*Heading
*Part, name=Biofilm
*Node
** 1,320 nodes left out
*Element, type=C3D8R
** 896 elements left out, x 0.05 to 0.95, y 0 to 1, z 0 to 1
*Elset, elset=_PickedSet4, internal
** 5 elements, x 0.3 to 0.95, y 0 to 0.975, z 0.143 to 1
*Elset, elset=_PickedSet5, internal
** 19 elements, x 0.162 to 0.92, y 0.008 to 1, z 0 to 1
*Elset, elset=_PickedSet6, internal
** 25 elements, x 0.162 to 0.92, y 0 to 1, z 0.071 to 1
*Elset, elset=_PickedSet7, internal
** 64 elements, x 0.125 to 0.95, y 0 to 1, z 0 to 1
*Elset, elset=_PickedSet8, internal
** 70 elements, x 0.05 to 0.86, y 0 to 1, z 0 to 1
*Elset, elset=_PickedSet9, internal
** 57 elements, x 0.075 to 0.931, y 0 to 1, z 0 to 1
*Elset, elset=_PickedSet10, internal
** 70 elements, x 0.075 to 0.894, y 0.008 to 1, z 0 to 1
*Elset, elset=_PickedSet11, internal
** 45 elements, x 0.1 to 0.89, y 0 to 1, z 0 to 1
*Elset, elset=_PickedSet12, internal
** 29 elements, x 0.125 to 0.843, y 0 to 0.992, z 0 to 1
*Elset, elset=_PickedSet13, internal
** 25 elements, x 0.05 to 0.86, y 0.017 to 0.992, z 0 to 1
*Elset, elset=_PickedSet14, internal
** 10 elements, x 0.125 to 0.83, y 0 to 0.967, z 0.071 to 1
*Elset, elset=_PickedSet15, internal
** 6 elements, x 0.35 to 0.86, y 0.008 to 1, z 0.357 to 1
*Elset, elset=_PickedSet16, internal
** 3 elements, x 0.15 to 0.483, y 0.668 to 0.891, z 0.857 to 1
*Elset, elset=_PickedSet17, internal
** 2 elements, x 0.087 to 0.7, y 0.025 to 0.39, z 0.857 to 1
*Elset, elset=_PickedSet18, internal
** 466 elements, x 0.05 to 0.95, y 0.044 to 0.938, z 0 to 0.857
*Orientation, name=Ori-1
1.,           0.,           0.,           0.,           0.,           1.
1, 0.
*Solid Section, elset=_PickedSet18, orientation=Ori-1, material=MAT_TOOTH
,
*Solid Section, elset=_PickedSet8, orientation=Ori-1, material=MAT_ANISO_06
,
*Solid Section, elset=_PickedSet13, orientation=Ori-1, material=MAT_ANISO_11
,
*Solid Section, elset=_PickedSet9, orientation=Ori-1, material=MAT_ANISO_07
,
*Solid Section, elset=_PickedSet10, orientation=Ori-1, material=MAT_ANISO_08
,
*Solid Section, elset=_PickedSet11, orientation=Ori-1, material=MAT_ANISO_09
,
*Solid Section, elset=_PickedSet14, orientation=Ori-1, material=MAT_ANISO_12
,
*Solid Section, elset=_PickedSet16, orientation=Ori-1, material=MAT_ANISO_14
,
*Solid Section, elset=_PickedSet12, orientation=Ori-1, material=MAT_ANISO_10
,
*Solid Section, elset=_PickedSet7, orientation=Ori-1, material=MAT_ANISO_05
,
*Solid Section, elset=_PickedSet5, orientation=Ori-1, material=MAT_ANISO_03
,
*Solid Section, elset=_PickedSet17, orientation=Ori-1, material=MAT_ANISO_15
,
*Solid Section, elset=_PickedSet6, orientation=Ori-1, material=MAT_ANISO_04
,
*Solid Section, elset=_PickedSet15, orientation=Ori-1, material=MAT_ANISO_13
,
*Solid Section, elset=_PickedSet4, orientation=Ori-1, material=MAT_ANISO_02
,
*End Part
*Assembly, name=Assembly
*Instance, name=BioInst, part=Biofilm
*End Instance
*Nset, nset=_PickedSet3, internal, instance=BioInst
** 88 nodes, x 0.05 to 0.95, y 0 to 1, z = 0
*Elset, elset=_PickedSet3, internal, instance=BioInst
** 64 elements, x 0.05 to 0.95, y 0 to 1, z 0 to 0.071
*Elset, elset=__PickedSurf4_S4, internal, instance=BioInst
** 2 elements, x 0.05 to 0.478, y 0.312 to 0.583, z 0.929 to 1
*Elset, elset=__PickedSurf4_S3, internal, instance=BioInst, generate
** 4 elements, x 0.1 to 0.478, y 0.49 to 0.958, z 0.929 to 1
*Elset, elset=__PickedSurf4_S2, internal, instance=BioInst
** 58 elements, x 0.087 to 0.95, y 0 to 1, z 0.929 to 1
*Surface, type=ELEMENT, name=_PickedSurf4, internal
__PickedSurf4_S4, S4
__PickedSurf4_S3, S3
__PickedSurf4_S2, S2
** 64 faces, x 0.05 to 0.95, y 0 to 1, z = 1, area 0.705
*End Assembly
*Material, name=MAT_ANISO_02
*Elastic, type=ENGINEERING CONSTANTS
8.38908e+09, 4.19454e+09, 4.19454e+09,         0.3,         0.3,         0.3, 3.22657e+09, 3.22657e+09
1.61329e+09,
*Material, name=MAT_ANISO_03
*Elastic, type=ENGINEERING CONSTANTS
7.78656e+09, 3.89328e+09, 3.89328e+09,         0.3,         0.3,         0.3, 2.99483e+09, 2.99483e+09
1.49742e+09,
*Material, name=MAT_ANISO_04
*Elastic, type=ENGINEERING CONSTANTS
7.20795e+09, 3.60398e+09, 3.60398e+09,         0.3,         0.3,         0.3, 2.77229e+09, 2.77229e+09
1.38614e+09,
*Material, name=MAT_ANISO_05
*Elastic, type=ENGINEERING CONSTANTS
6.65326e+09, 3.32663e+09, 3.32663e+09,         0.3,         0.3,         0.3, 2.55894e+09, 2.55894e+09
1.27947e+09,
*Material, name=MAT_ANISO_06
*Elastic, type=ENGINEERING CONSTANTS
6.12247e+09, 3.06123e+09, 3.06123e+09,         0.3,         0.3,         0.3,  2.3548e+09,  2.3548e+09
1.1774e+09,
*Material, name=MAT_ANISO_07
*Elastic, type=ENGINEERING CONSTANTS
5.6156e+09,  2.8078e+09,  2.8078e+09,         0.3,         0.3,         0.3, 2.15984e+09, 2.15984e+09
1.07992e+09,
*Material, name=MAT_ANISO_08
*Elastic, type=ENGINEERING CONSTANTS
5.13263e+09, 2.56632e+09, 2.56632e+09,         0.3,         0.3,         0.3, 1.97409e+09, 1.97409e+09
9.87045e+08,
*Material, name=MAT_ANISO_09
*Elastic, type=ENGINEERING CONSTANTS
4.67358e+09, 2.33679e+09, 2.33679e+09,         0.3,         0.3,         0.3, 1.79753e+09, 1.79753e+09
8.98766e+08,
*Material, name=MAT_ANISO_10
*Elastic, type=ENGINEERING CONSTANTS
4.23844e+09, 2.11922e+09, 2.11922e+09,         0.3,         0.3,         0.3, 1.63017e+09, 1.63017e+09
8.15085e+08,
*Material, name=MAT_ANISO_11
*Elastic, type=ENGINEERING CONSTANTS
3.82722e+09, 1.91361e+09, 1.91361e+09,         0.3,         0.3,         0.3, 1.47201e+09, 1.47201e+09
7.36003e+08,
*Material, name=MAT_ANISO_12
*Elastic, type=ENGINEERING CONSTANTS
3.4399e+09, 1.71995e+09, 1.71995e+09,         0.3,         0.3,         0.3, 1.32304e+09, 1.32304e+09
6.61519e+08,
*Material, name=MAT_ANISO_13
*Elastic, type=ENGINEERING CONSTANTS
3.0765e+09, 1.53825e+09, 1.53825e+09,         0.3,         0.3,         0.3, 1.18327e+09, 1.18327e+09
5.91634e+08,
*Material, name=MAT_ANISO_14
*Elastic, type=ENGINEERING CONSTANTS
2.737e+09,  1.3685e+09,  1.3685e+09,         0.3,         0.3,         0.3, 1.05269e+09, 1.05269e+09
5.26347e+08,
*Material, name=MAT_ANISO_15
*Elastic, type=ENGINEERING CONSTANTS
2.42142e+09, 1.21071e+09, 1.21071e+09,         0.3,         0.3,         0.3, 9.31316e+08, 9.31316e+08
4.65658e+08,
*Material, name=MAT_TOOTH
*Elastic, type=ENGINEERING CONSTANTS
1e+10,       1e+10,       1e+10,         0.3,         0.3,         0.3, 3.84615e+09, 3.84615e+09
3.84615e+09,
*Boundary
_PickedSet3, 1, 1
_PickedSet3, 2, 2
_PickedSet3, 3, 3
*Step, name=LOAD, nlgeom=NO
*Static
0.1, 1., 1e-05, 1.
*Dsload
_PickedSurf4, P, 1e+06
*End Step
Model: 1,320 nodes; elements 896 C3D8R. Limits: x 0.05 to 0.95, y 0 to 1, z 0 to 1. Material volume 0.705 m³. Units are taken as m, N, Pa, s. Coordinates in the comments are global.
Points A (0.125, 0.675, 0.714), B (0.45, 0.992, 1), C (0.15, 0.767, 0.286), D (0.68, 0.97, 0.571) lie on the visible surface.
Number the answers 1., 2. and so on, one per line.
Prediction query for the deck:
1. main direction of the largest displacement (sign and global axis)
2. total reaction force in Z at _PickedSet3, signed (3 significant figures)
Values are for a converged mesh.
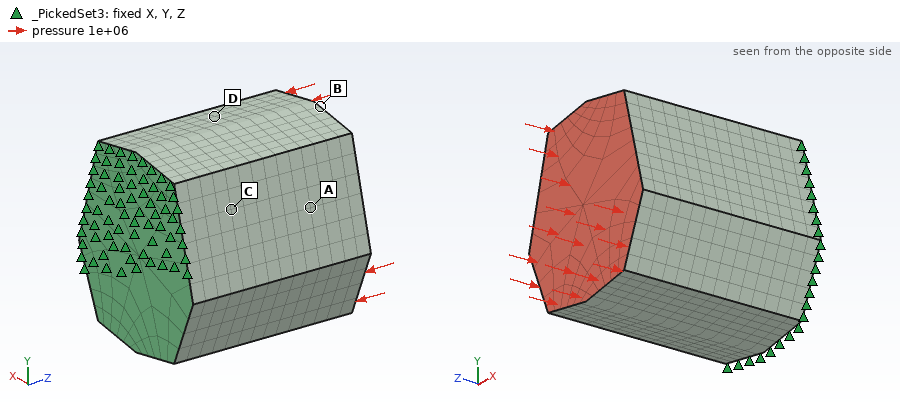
1. -Z
2. 7.05e+05 N
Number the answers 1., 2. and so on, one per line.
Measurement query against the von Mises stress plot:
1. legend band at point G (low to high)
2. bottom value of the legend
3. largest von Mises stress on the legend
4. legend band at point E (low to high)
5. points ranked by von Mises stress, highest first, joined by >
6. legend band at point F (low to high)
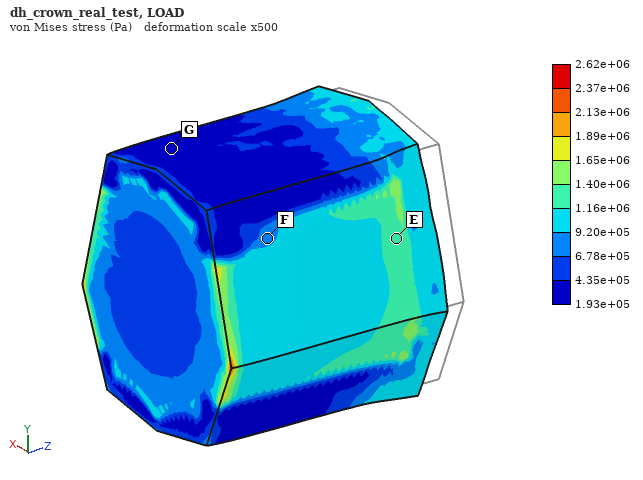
1. 1.93e+05 to 4.35e+05 Pa
2. 1.93e+05 Pa
3. 2.62e+06 Pa
4. 1.16e+06 to 1.40e+06 Pa
5. E > F > G
6. 6.78e+05 to 9.20e+05 Pa
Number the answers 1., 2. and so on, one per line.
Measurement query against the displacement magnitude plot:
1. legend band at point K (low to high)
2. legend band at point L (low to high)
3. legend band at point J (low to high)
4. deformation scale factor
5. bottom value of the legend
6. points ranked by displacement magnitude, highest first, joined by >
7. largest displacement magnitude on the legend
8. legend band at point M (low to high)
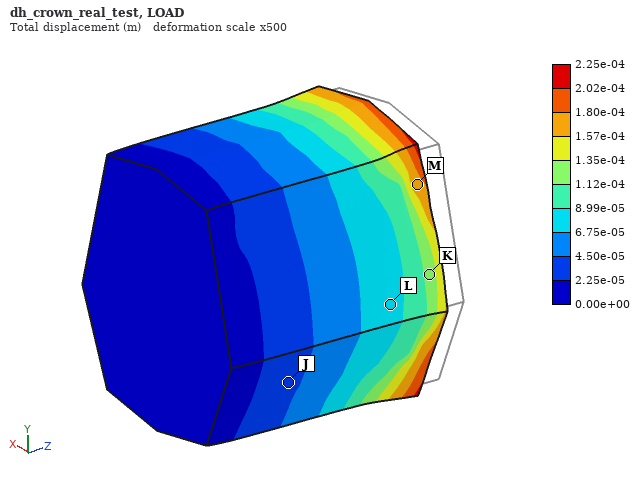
1. 1.12e-04 to 1.35e-04 m
2. 6.75e-05 to 8.99e-05 m
3. 2.25e-05 to 4.50e-05 m
4. 500
5. 0.00e+00 m
6. M > K > L > J
7. 2.25e-04 m
8. 1.57e-04 to 1.80e-04 m
